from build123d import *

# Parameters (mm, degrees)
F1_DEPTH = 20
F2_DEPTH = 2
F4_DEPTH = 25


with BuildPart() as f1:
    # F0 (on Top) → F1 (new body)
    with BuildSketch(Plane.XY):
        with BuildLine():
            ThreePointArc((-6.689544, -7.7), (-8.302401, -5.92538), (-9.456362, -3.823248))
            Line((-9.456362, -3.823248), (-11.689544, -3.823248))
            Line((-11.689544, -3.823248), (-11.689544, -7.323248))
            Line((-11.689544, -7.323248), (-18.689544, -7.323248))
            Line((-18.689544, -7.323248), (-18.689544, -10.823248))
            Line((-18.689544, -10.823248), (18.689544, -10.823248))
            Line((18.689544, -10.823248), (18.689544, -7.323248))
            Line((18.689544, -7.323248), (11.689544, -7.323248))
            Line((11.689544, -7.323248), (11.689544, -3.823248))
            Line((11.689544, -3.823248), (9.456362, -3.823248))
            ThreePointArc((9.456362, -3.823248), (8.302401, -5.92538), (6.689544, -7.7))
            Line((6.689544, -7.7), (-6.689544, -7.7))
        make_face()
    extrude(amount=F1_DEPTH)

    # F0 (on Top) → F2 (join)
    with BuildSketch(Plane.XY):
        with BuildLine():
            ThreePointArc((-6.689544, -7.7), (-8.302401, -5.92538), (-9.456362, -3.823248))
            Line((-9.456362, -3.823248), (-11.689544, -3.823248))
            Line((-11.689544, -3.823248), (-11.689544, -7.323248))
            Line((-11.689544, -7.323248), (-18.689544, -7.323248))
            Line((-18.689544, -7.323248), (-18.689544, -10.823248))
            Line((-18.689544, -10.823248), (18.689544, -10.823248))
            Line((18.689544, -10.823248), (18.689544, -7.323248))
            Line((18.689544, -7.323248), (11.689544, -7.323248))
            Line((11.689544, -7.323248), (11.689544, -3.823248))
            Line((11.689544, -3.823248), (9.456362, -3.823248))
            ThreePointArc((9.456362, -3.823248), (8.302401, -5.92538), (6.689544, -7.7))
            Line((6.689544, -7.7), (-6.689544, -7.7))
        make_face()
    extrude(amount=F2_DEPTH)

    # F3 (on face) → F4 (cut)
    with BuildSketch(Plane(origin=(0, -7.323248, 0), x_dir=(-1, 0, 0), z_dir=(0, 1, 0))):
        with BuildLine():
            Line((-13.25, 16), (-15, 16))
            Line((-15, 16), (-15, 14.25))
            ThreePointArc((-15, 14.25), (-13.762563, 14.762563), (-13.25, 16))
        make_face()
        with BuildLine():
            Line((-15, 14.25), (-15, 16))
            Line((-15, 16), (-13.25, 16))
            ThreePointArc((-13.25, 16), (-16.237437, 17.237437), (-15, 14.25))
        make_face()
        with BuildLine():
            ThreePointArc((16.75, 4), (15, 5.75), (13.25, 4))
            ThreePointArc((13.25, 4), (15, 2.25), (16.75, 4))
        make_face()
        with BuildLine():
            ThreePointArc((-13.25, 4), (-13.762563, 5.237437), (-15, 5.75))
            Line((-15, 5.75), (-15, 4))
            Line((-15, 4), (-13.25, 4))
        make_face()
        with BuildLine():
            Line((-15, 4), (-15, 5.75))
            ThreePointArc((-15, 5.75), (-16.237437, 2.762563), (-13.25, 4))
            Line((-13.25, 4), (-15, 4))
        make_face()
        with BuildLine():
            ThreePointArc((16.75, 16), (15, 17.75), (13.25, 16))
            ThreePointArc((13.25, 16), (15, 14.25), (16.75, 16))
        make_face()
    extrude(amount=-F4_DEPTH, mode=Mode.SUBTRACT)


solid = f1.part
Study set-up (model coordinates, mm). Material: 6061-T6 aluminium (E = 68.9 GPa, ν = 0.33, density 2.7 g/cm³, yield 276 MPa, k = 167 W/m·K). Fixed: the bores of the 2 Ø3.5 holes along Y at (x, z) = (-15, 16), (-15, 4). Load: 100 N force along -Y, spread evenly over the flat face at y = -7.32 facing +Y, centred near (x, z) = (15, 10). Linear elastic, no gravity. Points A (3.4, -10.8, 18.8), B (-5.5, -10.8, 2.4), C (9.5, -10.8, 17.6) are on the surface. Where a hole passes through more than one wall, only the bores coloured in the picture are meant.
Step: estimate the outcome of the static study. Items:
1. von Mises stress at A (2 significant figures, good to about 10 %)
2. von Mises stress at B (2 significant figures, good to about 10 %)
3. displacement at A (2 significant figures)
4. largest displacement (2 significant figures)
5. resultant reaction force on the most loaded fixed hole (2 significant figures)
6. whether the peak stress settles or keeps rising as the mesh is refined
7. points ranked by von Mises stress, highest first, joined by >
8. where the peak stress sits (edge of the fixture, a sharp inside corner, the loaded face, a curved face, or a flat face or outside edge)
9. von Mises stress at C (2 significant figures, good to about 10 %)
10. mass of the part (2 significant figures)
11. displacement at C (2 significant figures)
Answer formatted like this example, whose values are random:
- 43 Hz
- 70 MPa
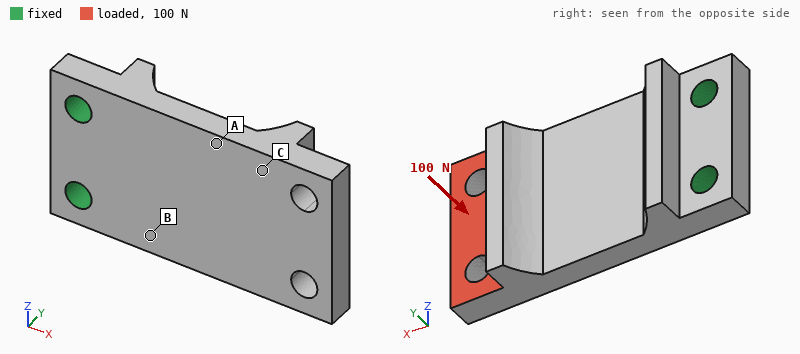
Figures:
- 37 MPa
- 58 MPa
- 0.073 mm
- 0.21 mm
- 55 N
- keeps rising
- B > A > C
- edge of the fixture
- 10 MPa
- 7.6 g
- 0.13 mm
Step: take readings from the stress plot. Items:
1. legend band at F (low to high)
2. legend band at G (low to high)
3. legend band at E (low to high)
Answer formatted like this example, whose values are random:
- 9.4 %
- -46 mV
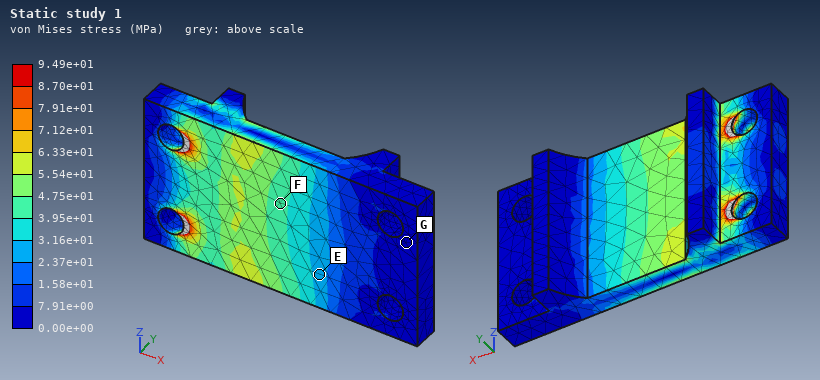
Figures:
- 3.95e+01 to 4.75e+01 MPa
- 0.00e+00 to 7.91e+00 MPa
- 2.37e+01 to 3.16e+01 MPa
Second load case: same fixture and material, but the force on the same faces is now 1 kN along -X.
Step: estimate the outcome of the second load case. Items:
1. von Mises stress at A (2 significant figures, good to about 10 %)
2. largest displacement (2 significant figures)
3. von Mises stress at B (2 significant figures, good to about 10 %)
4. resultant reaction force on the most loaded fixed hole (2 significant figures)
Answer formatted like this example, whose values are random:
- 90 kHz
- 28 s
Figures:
- 45 MPa
- 0.21 mm
- 38 MPa
- 500 N
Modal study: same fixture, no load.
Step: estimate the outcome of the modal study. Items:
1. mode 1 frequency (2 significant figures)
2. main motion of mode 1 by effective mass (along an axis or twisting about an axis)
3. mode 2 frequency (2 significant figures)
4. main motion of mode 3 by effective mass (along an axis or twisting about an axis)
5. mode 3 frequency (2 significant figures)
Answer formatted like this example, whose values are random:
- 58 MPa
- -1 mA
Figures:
- 2500 Hz
- along Y
- 8400 Hz
- along Z
- 11 kHz
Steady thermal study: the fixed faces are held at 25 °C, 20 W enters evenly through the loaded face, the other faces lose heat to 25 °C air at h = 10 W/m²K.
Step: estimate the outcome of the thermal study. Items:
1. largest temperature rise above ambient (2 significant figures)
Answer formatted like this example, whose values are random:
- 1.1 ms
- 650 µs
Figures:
- 54 K
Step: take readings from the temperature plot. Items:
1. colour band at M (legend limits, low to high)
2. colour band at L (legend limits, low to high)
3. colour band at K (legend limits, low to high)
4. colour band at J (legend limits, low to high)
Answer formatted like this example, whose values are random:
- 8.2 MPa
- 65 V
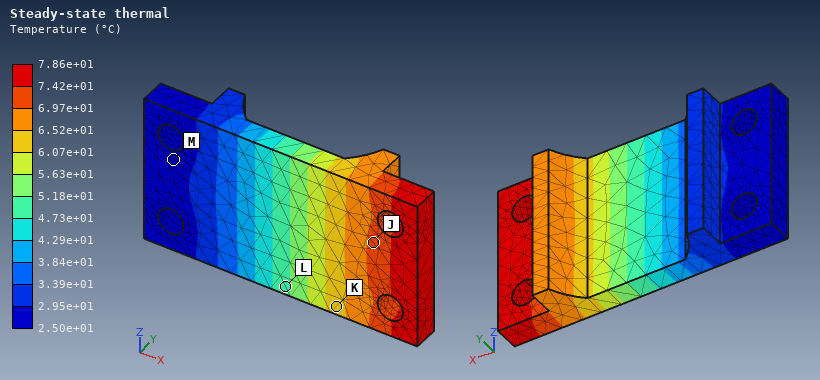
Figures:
- 2.50e+01 to 2.95e+01 °C
- 4.73e+01 to 5.18e+01 °C
- 6.07e+01 to 6.52e+01 °C
- 6.97e+01 to 7.42e+01 °C
